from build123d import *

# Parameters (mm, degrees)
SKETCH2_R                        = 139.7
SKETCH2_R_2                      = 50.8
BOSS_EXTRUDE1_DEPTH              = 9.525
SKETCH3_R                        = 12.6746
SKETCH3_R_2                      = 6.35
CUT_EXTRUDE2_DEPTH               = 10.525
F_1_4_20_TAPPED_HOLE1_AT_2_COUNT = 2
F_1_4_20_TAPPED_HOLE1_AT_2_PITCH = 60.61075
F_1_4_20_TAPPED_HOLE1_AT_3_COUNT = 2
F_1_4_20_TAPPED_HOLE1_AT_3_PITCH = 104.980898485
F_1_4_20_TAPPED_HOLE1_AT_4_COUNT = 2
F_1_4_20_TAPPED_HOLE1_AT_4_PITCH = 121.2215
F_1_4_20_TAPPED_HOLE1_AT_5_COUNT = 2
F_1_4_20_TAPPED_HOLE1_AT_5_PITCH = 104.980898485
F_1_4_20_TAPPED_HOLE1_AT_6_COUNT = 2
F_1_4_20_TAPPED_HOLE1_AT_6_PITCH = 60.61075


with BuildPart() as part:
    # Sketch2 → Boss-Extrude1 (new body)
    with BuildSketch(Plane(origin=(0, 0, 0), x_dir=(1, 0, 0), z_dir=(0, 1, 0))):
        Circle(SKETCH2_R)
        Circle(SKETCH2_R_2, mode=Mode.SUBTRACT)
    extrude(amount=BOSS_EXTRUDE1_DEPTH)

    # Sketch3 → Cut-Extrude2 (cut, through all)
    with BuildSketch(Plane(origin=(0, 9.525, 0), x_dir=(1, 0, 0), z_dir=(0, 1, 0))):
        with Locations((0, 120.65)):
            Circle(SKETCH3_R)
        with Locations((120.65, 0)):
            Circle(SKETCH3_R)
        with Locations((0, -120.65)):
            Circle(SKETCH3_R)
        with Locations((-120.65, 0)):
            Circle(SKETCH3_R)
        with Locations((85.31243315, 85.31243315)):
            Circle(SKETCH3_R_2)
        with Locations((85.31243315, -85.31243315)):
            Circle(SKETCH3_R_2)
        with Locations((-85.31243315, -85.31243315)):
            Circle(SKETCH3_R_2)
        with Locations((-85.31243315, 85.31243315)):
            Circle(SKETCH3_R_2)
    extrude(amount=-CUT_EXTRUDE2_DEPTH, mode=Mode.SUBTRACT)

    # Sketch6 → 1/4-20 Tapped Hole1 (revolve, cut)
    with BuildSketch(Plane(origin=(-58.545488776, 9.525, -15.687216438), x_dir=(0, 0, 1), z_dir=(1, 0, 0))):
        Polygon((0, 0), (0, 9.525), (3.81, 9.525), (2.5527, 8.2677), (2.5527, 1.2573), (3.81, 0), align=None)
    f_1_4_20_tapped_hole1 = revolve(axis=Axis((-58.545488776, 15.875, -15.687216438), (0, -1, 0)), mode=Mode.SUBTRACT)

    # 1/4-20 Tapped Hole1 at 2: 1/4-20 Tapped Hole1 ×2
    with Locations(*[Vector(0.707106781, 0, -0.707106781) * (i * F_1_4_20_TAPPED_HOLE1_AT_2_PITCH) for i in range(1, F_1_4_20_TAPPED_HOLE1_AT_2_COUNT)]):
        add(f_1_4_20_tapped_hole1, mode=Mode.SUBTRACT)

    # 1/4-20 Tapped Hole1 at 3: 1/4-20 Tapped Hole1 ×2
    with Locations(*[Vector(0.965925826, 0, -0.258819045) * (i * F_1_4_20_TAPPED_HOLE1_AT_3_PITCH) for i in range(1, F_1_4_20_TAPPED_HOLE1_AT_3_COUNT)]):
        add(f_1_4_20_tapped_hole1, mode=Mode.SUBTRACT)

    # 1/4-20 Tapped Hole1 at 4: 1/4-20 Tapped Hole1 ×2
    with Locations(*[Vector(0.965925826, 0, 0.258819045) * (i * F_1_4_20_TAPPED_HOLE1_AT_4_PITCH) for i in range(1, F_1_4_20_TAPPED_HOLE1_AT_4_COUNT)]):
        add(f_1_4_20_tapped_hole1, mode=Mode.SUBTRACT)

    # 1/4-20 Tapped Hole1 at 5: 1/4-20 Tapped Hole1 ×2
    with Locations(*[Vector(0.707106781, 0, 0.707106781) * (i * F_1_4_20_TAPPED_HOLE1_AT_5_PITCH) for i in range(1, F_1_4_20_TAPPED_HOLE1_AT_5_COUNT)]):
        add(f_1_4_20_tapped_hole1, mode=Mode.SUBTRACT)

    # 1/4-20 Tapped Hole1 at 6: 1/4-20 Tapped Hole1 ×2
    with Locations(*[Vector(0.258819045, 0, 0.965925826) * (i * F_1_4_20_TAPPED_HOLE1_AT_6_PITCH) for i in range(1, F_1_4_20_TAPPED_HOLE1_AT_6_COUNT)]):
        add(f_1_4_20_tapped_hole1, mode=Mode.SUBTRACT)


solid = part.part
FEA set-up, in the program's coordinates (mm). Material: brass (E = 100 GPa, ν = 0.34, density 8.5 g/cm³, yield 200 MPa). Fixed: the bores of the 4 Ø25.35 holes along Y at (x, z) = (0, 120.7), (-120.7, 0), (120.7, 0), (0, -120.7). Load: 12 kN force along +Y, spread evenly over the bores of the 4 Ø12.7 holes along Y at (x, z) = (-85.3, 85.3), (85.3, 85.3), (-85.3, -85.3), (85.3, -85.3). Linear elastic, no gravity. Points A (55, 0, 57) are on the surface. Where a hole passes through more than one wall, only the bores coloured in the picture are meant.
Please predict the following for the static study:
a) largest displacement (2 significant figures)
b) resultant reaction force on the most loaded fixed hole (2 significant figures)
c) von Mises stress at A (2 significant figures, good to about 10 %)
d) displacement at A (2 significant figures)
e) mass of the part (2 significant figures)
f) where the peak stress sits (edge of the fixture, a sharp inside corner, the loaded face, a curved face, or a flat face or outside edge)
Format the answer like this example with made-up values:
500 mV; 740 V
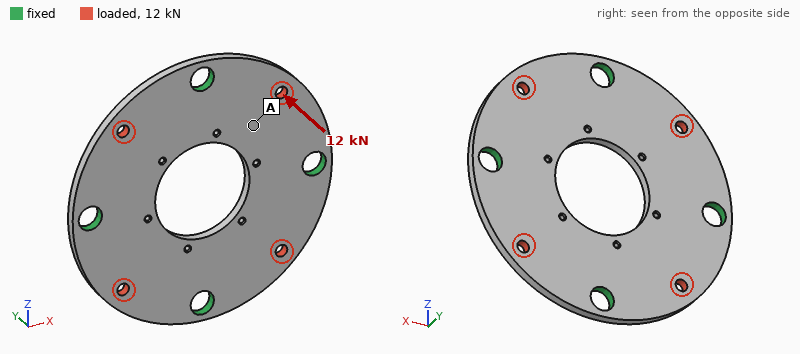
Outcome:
0.29 mm; 3.0 kN; 28 MPa; 0.060 mm; 4.1 kg; the loaded face
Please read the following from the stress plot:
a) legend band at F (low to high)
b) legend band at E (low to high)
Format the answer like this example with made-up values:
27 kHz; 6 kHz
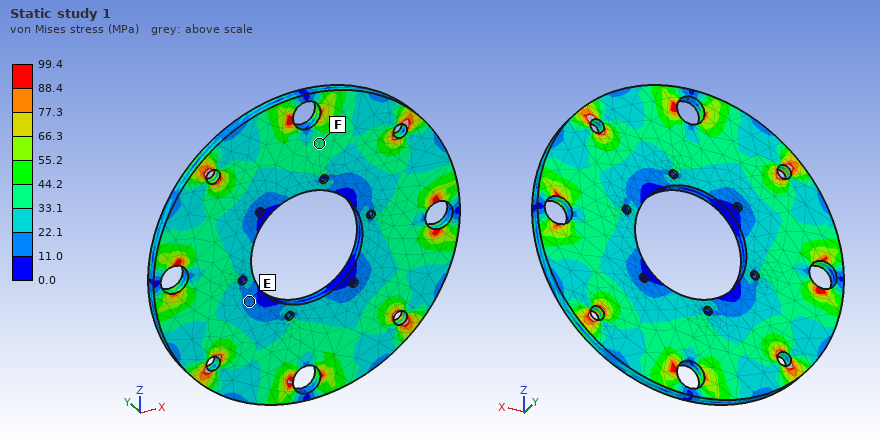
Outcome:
33.1 to 44.2 MPa; 11.0 to 22.1 MPa
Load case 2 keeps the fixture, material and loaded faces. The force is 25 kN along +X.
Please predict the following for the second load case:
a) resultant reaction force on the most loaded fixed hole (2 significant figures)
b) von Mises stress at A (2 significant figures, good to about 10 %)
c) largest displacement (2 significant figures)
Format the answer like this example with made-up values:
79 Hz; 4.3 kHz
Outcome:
8.1 kN; 3.5 MPa; 13 µm
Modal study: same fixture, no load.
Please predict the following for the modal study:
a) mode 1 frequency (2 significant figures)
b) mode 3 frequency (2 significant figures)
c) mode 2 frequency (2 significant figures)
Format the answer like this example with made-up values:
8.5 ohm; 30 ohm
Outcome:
1100 Hz; 1200 Hz; 1200 Hz
